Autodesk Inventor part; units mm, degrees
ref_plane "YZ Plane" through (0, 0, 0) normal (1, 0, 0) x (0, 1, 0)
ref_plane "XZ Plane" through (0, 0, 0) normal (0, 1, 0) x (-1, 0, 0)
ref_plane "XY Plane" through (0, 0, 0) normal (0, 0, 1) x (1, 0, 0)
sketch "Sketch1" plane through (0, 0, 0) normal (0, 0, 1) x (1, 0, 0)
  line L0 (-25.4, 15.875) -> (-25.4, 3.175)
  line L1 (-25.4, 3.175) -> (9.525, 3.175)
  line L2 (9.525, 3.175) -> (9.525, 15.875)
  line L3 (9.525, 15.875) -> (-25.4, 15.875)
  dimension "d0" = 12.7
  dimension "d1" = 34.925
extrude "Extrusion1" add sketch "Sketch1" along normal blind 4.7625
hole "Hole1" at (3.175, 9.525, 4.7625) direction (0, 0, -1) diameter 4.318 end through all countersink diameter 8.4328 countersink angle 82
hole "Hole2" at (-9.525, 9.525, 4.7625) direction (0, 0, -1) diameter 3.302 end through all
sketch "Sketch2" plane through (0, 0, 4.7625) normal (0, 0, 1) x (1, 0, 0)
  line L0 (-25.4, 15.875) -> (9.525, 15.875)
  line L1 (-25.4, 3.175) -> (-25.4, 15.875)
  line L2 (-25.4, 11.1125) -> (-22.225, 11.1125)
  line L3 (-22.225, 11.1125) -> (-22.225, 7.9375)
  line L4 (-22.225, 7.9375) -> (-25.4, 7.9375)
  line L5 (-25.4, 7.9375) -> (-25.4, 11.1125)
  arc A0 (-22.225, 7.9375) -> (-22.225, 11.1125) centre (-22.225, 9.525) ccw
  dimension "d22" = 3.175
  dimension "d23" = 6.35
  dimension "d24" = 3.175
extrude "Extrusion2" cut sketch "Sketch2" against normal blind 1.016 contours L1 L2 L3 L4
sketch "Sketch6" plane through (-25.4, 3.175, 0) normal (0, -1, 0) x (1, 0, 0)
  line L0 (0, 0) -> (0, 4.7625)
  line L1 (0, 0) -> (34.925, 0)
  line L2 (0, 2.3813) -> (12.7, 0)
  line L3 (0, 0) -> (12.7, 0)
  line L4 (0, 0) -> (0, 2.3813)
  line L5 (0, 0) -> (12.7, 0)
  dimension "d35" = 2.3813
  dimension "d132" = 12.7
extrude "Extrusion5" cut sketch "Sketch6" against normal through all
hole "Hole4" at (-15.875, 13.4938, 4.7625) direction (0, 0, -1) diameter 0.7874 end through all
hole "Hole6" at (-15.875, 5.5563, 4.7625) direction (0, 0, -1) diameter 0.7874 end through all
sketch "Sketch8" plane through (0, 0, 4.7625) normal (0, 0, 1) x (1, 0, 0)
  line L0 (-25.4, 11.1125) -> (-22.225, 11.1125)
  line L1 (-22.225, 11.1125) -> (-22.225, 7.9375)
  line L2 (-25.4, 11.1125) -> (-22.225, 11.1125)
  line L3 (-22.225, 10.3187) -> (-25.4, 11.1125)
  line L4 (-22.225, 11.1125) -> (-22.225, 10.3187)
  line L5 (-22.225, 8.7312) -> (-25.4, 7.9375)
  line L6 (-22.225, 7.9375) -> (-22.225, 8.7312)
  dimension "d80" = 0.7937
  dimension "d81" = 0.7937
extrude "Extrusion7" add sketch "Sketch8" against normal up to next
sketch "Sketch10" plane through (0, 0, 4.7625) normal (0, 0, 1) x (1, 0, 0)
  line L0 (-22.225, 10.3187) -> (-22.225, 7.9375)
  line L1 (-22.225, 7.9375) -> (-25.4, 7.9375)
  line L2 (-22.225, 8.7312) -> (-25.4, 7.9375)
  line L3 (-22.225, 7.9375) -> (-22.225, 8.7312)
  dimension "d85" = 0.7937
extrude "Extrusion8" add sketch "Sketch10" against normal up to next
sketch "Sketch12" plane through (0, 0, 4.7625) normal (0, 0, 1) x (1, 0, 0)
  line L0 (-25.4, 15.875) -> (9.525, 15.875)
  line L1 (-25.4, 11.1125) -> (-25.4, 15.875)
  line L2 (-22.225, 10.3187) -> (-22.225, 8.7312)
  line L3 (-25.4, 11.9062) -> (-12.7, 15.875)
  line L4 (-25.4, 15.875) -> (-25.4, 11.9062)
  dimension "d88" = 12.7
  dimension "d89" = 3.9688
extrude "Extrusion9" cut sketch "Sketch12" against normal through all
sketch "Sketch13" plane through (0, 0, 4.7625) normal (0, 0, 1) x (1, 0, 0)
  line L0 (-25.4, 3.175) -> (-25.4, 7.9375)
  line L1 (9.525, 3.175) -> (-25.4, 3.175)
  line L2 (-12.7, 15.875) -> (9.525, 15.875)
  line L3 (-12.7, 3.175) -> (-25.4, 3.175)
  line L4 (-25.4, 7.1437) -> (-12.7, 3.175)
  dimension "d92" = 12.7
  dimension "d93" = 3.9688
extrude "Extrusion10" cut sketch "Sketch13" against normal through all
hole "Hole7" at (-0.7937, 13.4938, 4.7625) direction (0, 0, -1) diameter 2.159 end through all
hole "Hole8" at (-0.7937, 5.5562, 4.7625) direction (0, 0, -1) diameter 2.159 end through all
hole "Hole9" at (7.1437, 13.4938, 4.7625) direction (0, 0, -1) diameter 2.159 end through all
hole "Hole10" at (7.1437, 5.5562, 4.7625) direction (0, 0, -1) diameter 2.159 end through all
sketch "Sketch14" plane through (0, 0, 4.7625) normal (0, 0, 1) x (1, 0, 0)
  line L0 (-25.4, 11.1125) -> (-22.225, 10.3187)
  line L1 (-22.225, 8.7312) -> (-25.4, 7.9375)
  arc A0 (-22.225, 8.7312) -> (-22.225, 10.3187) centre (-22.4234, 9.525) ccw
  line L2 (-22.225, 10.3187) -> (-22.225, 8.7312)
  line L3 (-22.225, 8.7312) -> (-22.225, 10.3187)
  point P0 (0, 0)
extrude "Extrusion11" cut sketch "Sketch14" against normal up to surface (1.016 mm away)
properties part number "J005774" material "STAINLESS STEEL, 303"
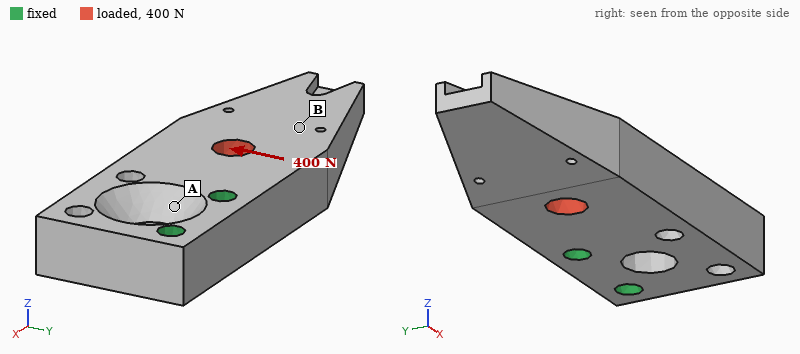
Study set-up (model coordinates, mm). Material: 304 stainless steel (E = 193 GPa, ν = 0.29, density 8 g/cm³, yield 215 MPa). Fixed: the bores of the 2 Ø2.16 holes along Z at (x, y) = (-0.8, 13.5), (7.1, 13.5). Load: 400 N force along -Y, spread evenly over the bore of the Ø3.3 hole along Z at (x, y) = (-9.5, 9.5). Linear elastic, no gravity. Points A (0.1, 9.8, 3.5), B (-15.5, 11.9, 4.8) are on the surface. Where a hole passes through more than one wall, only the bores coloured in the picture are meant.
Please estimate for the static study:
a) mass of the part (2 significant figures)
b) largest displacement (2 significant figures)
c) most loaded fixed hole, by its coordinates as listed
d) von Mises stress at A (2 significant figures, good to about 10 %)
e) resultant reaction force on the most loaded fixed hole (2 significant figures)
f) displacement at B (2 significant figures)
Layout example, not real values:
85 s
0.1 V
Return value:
12 g
10 µm
(-0.8, 13.5)
26 MPa
640 N
6.4 µm
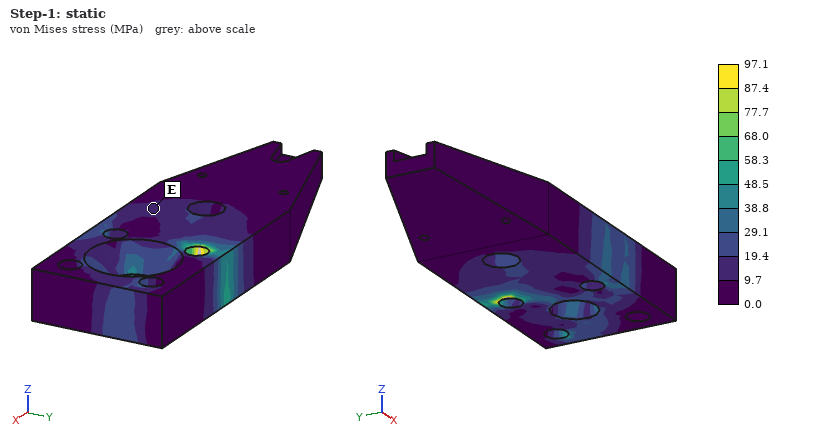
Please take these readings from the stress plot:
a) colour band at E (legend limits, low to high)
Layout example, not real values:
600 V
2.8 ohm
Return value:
9.7 to 19.4 MPa
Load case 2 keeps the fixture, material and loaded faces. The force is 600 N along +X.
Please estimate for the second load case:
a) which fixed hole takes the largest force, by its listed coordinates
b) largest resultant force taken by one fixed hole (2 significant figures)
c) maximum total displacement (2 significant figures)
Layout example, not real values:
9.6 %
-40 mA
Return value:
(-0.8, 13.5)
500 N
5.7 µm
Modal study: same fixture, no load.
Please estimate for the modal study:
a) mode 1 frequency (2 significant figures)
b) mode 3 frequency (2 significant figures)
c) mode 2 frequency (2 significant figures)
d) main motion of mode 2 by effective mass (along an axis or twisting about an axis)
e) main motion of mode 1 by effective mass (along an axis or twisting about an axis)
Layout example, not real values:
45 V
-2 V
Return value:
7500 Hz
20 kHz
12 kHz
along Y
along Z
